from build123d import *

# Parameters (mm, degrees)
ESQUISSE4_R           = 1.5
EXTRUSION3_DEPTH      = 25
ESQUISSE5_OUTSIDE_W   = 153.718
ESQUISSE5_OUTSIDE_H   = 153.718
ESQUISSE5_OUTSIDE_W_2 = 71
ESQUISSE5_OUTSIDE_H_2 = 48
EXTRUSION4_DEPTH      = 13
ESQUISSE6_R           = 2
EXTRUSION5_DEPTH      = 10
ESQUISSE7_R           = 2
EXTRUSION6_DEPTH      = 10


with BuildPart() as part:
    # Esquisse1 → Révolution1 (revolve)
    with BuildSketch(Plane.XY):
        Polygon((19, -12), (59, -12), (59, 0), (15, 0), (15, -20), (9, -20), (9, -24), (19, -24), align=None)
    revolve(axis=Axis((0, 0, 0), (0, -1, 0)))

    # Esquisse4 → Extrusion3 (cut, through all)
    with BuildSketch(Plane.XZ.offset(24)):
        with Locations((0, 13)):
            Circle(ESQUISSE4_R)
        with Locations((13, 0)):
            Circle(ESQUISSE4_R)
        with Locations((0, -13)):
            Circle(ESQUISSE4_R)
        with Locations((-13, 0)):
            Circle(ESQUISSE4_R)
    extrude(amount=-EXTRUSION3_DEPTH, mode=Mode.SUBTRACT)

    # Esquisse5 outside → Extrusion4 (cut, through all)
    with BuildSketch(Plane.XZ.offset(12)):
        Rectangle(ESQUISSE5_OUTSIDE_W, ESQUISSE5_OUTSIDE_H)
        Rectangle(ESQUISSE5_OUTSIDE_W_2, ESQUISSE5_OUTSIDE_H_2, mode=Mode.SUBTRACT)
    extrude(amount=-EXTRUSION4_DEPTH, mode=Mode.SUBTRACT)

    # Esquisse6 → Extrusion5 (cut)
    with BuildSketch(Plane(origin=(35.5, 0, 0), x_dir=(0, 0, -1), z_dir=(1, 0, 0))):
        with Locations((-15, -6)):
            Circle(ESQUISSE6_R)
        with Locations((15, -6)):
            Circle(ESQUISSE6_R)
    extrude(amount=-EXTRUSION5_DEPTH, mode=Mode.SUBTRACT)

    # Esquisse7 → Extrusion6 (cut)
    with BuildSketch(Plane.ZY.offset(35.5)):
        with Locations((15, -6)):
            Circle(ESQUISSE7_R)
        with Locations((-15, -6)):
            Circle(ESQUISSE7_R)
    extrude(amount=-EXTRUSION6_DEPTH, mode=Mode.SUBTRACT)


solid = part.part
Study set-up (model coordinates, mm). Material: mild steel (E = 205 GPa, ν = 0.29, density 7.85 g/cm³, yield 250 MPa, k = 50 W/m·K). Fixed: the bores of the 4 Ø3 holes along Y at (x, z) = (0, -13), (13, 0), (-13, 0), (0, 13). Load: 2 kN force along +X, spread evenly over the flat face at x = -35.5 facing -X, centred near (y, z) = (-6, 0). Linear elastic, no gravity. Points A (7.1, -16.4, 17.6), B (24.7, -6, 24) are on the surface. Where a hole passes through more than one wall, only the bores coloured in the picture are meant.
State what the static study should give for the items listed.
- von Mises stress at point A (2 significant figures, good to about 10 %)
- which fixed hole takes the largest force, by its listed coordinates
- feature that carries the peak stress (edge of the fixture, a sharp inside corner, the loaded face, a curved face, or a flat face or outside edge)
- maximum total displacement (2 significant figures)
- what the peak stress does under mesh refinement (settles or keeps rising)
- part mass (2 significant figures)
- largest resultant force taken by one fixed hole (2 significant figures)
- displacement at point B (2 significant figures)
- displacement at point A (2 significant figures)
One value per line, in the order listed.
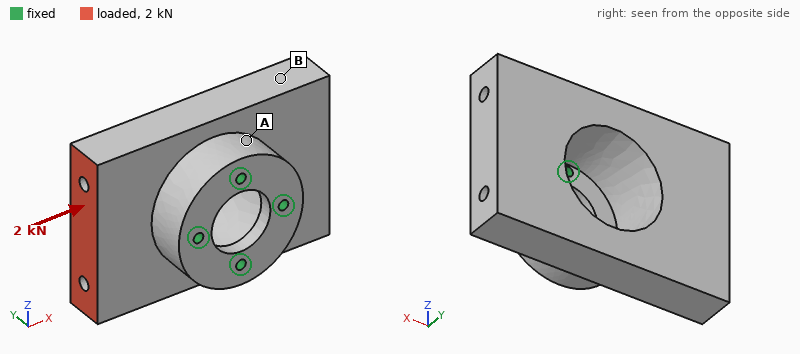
12 MPa
(-13, 0)
edge of the fixture
9.3 µm
keeps rising
300 g
1.0 kN
5.8 µm
2.3 µm
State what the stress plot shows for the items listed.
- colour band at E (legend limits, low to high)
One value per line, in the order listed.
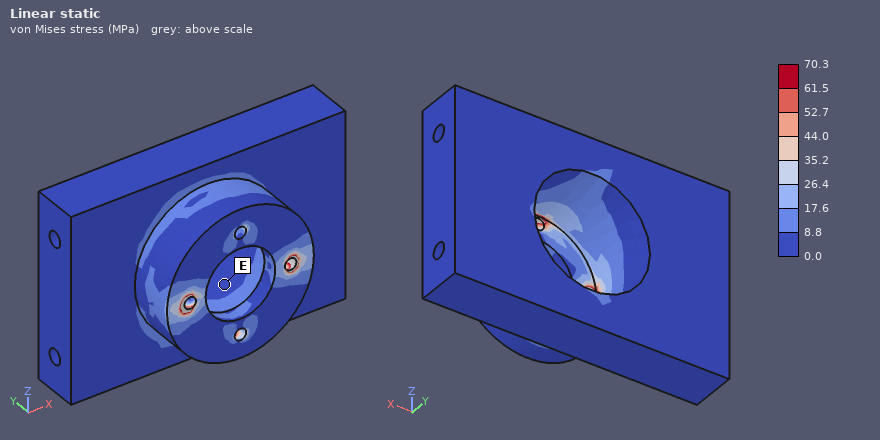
0.0 to 8.8 MPa
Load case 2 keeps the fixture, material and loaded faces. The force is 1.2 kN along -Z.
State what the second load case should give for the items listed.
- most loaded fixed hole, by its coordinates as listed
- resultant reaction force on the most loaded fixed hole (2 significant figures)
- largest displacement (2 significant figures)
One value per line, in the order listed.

(-13, 0)
1.3 kN
8.1 µm
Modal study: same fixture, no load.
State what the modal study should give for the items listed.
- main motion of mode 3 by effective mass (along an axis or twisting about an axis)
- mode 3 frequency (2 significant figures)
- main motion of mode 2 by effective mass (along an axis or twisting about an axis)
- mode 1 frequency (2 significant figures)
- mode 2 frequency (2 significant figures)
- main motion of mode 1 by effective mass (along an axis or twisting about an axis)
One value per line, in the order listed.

twisting about Y
8000 Hz
along Z
4700 Hz
5600 Hz
along X
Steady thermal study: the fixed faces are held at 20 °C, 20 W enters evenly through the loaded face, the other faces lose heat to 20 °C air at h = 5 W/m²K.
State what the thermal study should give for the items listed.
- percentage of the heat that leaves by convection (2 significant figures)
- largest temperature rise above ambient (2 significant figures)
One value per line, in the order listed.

4.9 %
39 K
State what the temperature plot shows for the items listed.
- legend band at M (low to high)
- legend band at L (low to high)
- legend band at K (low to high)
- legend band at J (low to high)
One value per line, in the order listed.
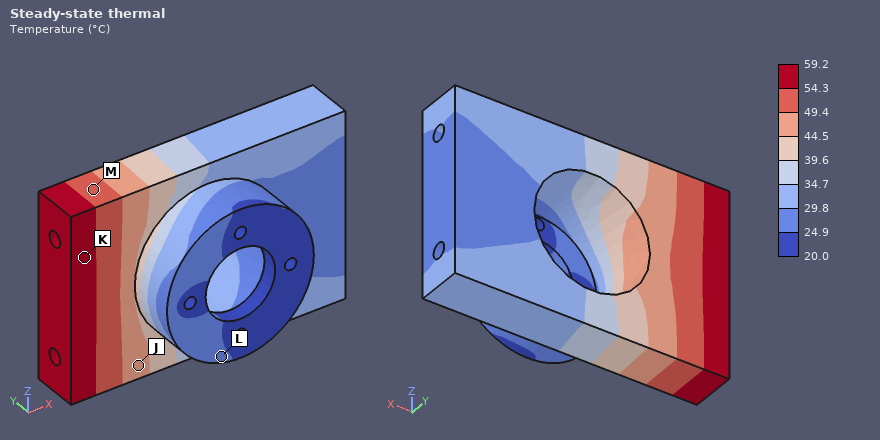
49.4 to 54.3 °C
24.9 to 29.8 °C
54.3 to 59.2 °C
44.5 to 49.4 °C
